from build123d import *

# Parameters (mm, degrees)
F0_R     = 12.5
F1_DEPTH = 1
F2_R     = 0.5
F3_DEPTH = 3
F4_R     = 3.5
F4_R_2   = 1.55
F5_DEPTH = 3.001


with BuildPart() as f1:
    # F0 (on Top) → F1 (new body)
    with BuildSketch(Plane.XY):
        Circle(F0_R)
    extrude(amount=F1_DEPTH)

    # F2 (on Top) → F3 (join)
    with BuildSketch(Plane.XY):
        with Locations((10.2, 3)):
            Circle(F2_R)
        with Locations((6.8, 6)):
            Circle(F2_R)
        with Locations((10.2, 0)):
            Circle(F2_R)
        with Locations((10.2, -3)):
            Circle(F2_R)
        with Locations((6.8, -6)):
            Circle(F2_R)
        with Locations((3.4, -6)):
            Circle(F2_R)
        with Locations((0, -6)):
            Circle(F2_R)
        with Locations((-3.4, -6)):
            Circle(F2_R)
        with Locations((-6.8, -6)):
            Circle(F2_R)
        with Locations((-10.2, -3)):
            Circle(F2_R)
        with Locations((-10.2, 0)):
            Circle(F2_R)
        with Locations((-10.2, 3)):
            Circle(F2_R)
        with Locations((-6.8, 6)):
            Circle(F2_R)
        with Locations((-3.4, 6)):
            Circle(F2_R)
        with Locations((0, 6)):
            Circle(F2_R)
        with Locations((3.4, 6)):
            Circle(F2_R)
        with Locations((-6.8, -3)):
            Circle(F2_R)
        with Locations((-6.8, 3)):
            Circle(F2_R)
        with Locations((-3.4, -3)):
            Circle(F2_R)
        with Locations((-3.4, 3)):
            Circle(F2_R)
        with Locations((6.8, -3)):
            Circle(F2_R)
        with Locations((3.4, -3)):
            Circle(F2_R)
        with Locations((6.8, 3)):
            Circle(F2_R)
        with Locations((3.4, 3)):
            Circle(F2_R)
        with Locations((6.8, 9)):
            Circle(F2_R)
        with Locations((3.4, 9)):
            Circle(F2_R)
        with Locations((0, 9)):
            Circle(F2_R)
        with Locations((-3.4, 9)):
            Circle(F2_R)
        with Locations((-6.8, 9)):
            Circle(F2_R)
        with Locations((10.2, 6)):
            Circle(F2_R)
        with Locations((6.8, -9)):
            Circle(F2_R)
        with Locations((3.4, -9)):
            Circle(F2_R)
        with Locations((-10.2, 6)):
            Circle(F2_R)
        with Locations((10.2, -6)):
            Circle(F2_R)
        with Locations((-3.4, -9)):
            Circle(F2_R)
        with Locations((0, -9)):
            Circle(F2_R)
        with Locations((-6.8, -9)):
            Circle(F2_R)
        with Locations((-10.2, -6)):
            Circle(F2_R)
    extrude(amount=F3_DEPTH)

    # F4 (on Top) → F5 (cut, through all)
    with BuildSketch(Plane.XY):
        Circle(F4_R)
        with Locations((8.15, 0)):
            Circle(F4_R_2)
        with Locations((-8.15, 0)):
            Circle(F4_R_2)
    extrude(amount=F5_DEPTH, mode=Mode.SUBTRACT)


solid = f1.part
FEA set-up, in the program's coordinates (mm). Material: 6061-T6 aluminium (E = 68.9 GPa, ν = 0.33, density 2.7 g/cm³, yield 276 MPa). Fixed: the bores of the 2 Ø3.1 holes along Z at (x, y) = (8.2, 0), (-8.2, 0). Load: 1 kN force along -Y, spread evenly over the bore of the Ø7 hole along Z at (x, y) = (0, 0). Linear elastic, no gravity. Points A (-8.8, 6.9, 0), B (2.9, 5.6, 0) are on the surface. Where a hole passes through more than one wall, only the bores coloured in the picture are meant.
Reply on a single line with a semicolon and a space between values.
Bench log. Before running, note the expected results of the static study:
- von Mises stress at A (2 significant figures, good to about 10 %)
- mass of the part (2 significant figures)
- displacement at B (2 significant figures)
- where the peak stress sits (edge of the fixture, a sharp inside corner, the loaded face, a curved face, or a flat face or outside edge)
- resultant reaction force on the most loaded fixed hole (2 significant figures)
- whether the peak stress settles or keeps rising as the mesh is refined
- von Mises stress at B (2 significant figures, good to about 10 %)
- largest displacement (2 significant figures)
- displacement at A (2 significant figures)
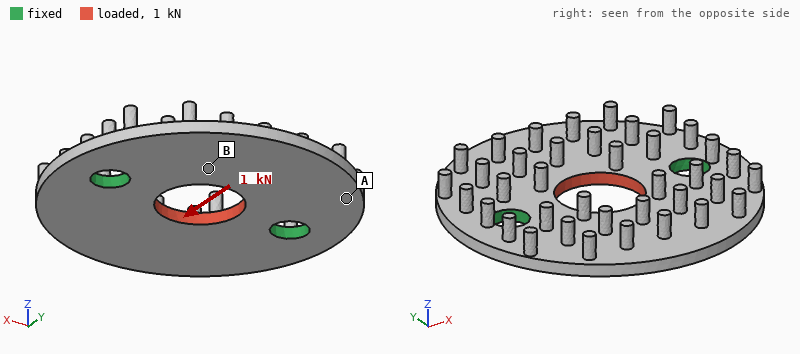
17 MPa; 1.3 g; 6.0 µm; edge of the fixture; 500 N; keeps rising; 37 MPa; 8.4 µm; 2.1 µm
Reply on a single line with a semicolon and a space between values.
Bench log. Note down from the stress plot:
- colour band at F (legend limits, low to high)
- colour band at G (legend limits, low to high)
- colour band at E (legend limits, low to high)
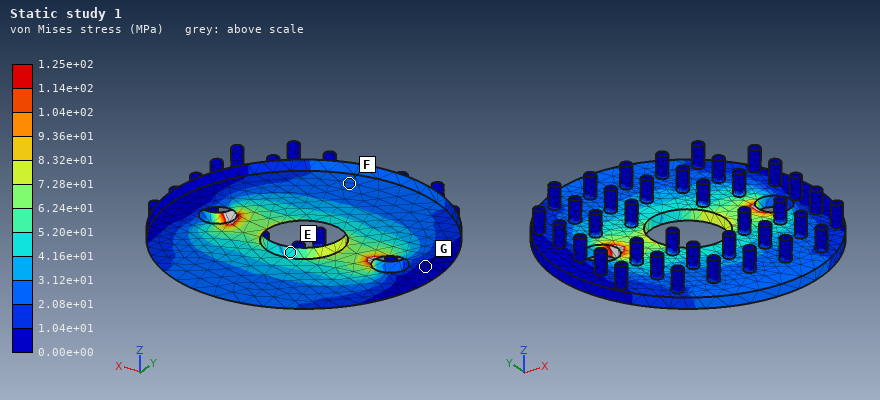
2.08e+01 to 3.12e+01 MPa; 0.00e+00 to 1.04e+01 MPa; 4.16e+01 to 5.20e+01 MPa
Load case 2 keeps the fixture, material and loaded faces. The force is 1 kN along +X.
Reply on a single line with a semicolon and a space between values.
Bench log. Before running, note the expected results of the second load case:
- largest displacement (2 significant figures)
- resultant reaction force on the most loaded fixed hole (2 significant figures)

6.7 µm; 500 N
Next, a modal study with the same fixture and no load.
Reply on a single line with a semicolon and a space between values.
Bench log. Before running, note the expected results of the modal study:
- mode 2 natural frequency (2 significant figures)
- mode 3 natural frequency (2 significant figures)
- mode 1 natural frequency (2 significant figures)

6500 Hz; 15 kHz; 6300 Hz
